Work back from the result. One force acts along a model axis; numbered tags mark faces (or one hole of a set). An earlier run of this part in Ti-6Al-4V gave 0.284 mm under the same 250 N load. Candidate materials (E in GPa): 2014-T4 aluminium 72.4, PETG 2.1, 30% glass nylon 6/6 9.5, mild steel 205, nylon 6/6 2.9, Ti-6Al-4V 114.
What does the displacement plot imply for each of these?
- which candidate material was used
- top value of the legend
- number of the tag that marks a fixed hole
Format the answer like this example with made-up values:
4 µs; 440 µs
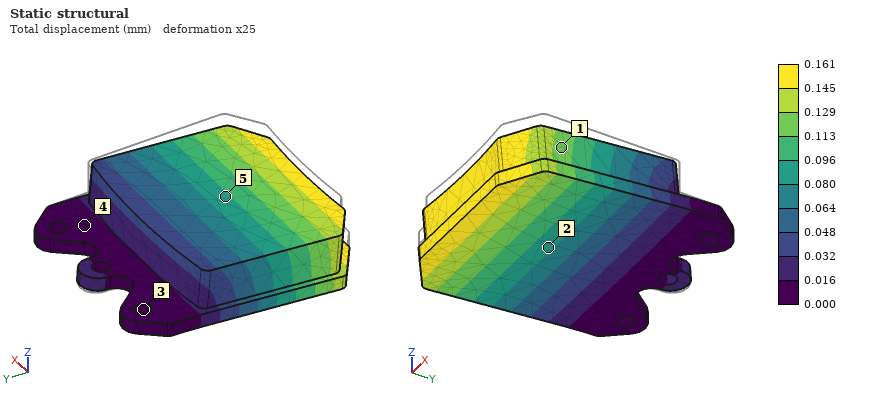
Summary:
mild steel; 0.161 mm; 3
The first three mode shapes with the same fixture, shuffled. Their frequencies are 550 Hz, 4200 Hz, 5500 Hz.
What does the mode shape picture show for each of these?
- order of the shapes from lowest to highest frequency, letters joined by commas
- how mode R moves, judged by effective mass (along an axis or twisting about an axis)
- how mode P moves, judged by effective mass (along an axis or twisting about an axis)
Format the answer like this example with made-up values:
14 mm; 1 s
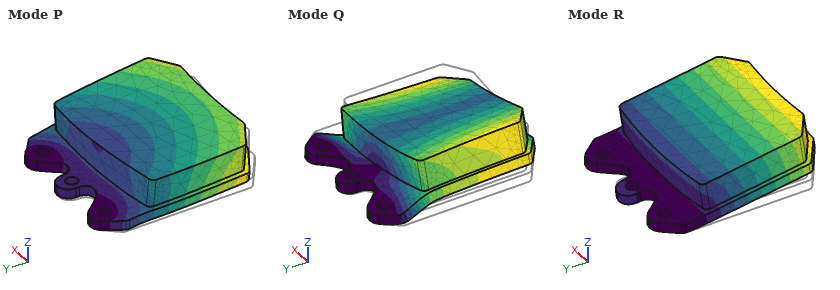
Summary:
R, Q, P; along Z; along X
